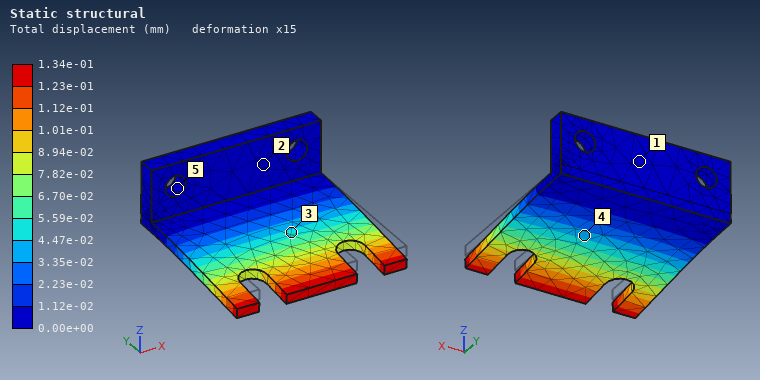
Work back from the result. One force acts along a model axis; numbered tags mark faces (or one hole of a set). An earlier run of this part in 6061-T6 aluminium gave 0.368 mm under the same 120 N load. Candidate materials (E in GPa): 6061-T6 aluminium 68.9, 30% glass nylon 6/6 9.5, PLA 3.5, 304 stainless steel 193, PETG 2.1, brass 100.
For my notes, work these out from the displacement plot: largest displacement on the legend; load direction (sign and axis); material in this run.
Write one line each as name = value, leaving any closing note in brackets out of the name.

largest displacement on the legend = 1.34e-01 mm
load direction = -Z
material in this run = 304 stainless steel
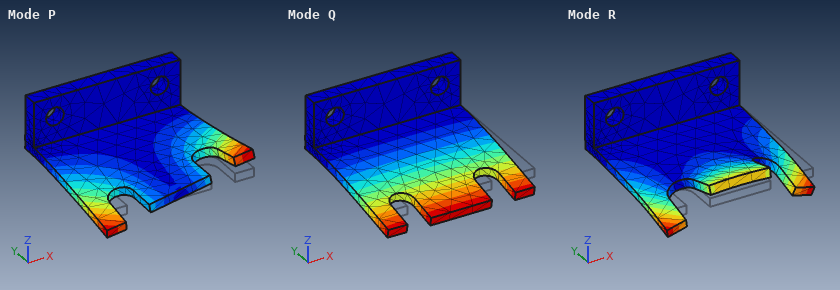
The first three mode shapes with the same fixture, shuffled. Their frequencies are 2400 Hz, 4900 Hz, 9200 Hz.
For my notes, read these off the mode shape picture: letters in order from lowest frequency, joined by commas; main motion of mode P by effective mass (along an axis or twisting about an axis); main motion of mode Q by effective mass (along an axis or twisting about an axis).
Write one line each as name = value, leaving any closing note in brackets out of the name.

letters in order from lowest frequency, joined by commas = Q, P, R
main motion of mode P by effective mass = twisting about Y
main motion of mode Q by effective mass = along Z
